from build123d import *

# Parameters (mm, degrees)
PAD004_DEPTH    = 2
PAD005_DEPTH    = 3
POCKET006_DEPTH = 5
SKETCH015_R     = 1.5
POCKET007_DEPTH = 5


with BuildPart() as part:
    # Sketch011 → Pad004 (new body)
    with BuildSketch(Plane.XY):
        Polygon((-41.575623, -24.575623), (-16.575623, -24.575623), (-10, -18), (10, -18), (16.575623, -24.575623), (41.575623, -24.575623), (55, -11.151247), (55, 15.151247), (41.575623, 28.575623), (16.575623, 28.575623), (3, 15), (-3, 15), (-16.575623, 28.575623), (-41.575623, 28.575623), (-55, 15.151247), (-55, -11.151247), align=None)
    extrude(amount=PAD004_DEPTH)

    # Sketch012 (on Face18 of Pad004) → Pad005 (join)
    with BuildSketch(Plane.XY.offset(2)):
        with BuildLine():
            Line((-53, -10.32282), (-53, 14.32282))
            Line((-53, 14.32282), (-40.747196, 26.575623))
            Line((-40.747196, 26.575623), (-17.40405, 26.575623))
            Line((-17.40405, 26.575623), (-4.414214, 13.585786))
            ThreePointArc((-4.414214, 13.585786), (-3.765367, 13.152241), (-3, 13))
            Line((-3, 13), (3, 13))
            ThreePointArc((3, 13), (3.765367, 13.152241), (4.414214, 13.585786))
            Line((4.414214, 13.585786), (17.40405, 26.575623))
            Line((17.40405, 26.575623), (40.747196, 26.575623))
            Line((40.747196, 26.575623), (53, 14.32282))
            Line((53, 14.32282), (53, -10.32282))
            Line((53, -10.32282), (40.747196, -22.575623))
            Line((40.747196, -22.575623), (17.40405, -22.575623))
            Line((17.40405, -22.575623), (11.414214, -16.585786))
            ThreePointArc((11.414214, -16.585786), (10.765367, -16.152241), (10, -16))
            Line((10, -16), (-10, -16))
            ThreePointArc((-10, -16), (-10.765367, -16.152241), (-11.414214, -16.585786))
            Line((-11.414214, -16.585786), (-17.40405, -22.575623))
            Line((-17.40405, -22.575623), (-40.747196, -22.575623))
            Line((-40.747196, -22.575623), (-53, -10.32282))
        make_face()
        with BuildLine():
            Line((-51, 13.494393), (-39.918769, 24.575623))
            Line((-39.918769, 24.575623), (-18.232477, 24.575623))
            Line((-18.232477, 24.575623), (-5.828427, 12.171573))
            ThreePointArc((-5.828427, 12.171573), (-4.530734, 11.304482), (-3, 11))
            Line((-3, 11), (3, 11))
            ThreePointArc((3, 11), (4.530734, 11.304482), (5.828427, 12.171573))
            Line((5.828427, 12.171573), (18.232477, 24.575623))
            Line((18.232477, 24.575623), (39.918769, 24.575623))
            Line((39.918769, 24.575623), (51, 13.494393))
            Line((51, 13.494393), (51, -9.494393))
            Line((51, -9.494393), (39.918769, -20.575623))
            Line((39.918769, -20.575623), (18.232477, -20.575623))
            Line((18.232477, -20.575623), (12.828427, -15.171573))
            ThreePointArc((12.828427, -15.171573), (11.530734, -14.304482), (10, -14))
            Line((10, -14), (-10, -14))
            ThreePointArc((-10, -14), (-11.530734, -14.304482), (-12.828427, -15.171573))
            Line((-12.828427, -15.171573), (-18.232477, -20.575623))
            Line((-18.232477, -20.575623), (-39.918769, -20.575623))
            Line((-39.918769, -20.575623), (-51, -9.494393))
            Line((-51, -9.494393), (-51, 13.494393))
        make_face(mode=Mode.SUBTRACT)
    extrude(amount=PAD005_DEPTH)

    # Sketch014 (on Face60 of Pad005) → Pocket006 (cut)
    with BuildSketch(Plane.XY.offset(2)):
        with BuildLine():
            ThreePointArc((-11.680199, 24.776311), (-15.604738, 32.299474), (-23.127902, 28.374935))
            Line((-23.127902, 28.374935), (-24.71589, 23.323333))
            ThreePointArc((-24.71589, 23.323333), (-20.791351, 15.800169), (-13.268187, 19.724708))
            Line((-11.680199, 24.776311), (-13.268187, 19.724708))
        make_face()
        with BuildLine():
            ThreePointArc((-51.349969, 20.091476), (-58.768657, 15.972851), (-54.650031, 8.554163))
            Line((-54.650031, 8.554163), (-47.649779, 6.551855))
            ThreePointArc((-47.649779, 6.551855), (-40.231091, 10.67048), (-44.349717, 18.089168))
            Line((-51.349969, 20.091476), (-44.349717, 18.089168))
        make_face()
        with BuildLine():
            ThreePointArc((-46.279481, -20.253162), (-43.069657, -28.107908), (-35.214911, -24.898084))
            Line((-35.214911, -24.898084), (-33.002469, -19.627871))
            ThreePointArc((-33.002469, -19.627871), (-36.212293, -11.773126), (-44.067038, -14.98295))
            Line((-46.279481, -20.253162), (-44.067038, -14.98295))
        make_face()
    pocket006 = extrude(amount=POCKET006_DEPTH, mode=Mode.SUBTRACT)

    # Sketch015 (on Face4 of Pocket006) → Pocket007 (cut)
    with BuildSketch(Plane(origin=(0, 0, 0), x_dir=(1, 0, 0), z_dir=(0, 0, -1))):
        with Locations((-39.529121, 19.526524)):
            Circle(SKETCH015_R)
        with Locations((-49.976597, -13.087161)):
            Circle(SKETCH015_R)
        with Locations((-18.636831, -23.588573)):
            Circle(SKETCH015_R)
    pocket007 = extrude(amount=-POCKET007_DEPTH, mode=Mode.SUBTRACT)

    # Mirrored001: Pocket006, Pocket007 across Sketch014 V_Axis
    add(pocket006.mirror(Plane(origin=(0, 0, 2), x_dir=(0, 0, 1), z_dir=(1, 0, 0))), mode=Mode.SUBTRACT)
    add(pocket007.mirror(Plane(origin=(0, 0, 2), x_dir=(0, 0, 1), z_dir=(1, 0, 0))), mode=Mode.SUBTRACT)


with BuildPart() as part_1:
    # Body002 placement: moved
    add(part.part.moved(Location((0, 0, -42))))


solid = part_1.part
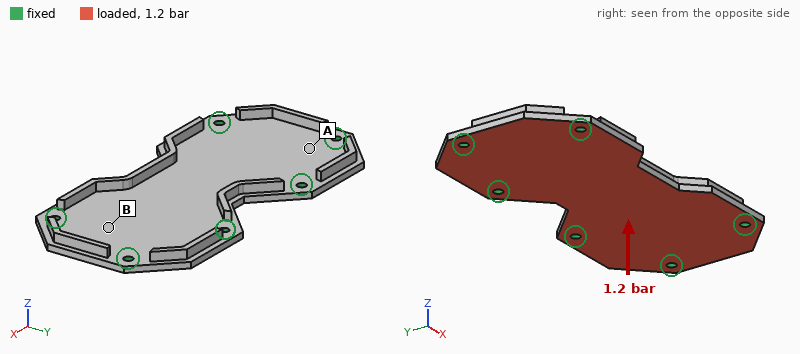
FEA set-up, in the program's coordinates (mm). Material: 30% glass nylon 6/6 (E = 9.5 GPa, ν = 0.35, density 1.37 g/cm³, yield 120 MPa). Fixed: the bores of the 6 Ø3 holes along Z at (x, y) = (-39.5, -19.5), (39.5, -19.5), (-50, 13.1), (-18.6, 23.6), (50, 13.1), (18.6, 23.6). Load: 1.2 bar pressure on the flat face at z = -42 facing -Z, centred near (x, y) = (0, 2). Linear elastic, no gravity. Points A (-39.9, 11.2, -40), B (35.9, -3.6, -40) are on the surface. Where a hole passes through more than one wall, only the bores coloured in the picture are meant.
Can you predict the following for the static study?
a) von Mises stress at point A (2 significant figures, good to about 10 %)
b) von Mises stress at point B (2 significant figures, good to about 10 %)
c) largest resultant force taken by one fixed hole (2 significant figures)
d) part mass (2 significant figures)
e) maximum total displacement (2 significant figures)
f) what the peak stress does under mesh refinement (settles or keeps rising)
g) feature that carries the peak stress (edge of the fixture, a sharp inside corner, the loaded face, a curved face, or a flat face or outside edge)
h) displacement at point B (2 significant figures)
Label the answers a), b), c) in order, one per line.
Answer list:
a) 7.1 MPa
b) 15 MPa
c) 140 N
d) 15 g
e) 0.90 mm
f) keeps rising
g) edge of the fixture
h) 0.19 mm
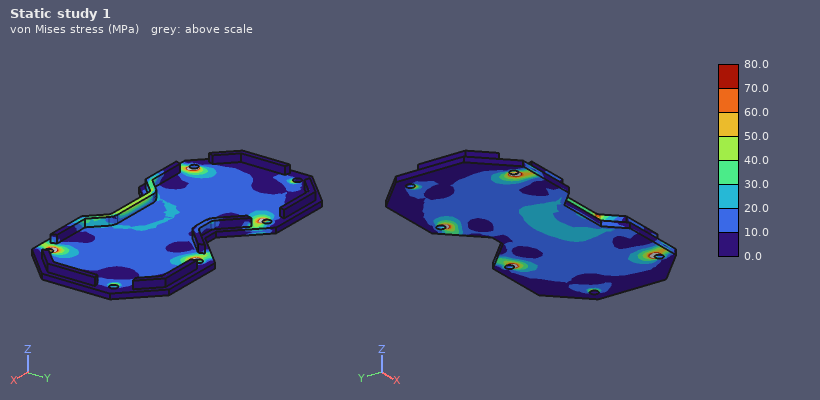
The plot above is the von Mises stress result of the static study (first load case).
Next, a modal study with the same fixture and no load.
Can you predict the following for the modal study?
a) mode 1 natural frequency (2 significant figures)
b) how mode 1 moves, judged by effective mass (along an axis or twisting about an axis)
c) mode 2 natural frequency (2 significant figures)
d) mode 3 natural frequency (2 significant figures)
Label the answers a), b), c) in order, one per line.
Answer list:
a) 1300 Hz
b) along Z
c) 2800 Hz
d) 2900 Hz
